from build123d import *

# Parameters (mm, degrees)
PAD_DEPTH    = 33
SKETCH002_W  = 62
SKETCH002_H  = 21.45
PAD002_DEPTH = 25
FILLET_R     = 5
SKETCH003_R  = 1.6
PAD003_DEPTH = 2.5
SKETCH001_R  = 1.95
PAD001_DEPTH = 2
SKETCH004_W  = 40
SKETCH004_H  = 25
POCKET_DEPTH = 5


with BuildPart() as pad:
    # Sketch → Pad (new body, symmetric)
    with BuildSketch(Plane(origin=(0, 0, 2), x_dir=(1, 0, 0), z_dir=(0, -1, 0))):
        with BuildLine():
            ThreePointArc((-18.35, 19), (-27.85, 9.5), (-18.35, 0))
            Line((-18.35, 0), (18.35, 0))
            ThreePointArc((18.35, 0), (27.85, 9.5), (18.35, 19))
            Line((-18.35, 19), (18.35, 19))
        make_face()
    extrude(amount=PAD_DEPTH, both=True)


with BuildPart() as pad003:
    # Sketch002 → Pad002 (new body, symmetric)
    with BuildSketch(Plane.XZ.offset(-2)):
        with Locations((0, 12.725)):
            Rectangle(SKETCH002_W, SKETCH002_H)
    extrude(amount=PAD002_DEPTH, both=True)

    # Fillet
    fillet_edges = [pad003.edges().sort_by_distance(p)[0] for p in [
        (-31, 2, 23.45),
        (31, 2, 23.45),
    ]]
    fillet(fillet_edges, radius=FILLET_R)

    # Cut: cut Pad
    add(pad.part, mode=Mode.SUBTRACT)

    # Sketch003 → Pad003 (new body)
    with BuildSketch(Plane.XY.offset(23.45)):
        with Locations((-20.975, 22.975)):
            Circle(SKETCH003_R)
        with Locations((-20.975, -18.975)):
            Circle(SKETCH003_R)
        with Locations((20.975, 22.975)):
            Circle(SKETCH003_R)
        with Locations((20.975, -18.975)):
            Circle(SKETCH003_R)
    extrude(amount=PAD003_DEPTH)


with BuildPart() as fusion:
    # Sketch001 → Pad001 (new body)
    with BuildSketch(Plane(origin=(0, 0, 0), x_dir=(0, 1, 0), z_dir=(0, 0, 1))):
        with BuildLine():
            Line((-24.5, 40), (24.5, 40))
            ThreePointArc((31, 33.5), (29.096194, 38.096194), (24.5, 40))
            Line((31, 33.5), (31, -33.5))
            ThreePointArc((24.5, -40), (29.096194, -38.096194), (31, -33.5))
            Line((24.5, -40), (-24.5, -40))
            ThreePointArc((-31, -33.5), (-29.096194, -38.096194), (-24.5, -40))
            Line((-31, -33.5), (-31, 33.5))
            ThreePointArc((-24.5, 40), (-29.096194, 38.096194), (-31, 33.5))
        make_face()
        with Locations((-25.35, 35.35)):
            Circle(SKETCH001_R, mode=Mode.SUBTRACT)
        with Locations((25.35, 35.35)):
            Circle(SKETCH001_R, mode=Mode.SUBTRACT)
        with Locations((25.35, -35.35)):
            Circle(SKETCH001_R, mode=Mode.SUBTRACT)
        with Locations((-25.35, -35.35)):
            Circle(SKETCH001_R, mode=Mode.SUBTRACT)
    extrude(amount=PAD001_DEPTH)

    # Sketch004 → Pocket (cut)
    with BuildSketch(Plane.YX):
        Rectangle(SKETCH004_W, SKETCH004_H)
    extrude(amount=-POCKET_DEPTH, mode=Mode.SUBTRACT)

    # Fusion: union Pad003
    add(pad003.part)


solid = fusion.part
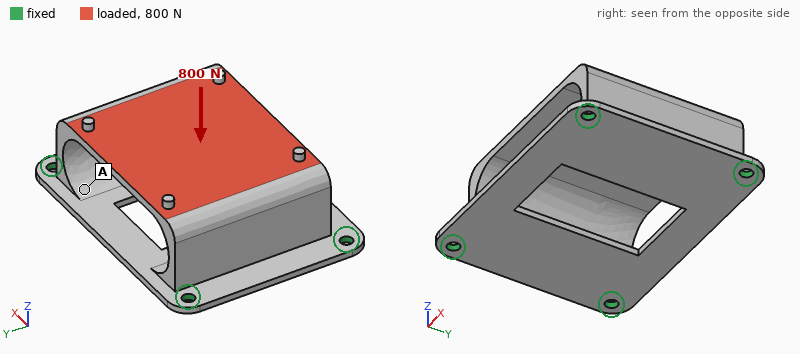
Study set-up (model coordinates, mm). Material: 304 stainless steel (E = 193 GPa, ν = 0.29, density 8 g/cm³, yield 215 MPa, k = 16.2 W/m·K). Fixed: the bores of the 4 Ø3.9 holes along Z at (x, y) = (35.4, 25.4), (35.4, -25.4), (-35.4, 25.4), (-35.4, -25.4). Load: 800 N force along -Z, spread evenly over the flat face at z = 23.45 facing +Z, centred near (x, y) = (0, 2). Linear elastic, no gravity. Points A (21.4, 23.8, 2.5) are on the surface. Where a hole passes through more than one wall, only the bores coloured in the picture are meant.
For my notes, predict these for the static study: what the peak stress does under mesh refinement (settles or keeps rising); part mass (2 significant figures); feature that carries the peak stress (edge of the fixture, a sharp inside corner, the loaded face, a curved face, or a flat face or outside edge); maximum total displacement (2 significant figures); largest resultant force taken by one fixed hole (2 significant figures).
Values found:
keeps rising
200 g
edge of the fixture
26 µm
280 N
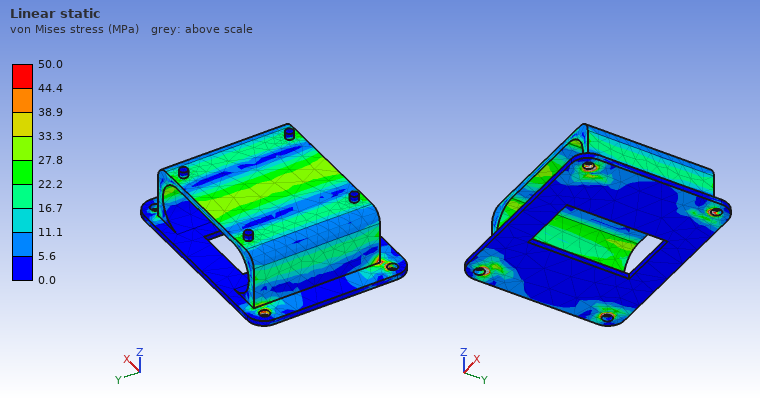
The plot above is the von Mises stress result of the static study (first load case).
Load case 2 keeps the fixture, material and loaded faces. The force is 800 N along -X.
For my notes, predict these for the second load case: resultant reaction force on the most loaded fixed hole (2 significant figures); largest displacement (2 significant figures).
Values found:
270 N
45 µm
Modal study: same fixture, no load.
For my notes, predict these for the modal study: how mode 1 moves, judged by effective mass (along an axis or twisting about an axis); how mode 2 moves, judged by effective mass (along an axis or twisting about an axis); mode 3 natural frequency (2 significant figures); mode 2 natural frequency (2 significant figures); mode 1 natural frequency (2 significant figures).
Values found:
along X
along Z
4500 Hz
4000 Hz
2300 Hz
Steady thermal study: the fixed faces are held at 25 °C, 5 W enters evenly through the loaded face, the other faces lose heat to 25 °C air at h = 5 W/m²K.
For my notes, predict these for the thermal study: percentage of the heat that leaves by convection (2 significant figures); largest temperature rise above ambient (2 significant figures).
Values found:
29 %
40 K
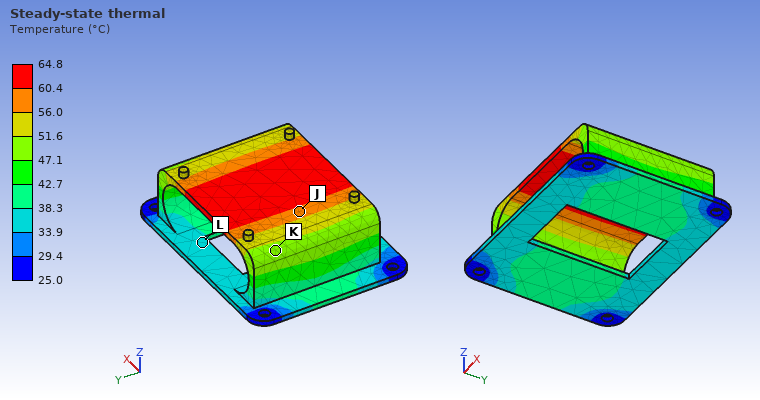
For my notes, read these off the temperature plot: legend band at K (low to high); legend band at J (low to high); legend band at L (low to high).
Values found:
47.1 to 51.6 °C
56.0 to 60.4 °C
33.9 to 38.3 °C
